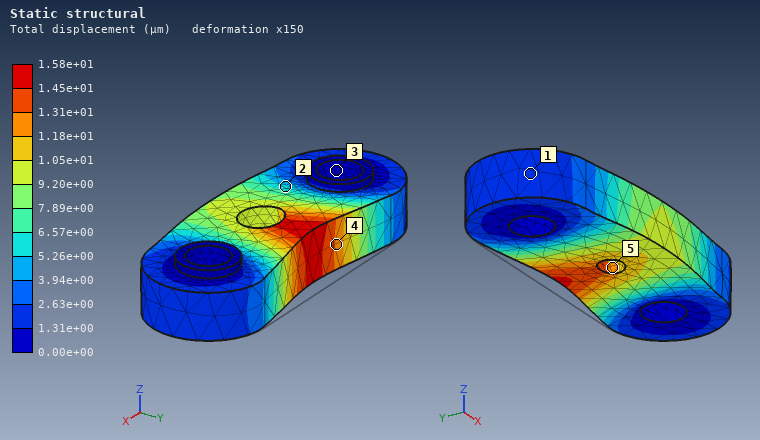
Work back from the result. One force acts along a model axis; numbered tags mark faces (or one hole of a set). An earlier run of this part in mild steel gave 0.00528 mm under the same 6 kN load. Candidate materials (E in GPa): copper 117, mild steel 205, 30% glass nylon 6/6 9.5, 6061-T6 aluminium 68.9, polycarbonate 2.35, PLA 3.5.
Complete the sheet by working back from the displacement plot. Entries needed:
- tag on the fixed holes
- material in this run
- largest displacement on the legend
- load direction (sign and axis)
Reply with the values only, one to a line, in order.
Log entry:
3
6061-T6 aluminium
1.58e+01 µm
-Y
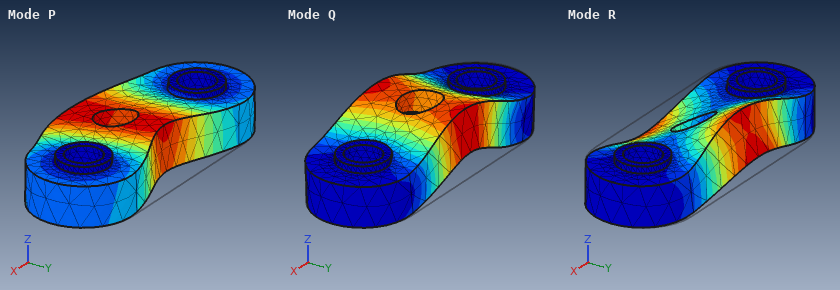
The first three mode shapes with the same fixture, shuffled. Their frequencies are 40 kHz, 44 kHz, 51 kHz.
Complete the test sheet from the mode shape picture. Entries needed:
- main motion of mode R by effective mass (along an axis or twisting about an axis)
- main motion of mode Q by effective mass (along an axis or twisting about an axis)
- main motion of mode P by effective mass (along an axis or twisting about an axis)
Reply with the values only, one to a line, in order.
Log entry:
twisting about X
along Z
along Y
